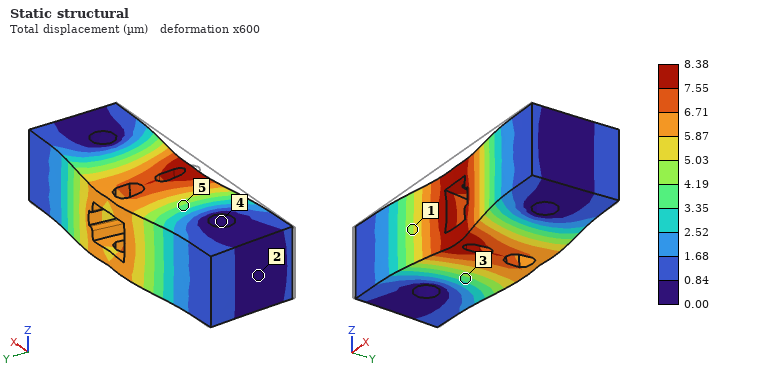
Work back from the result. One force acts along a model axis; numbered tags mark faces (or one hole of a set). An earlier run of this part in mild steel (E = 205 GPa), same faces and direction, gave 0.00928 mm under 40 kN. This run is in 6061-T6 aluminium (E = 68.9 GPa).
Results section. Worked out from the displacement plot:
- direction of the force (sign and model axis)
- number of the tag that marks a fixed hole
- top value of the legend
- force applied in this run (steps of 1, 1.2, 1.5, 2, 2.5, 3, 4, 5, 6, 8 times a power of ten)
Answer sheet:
+Y
4
8.38 µm
12 kN
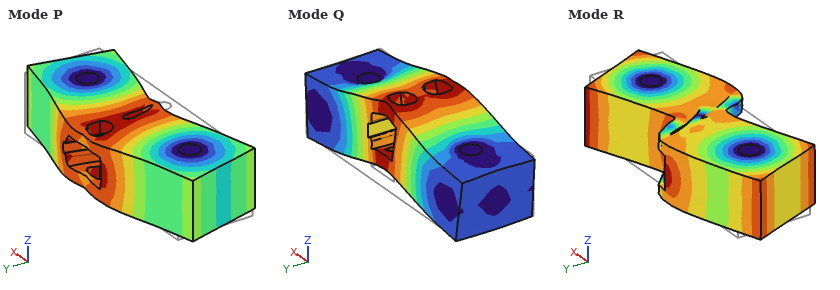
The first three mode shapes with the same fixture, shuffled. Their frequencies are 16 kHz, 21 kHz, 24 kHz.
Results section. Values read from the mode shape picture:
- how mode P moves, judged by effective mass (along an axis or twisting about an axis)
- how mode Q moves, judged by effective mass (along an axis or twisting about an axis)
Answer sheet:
along Y
along Z
